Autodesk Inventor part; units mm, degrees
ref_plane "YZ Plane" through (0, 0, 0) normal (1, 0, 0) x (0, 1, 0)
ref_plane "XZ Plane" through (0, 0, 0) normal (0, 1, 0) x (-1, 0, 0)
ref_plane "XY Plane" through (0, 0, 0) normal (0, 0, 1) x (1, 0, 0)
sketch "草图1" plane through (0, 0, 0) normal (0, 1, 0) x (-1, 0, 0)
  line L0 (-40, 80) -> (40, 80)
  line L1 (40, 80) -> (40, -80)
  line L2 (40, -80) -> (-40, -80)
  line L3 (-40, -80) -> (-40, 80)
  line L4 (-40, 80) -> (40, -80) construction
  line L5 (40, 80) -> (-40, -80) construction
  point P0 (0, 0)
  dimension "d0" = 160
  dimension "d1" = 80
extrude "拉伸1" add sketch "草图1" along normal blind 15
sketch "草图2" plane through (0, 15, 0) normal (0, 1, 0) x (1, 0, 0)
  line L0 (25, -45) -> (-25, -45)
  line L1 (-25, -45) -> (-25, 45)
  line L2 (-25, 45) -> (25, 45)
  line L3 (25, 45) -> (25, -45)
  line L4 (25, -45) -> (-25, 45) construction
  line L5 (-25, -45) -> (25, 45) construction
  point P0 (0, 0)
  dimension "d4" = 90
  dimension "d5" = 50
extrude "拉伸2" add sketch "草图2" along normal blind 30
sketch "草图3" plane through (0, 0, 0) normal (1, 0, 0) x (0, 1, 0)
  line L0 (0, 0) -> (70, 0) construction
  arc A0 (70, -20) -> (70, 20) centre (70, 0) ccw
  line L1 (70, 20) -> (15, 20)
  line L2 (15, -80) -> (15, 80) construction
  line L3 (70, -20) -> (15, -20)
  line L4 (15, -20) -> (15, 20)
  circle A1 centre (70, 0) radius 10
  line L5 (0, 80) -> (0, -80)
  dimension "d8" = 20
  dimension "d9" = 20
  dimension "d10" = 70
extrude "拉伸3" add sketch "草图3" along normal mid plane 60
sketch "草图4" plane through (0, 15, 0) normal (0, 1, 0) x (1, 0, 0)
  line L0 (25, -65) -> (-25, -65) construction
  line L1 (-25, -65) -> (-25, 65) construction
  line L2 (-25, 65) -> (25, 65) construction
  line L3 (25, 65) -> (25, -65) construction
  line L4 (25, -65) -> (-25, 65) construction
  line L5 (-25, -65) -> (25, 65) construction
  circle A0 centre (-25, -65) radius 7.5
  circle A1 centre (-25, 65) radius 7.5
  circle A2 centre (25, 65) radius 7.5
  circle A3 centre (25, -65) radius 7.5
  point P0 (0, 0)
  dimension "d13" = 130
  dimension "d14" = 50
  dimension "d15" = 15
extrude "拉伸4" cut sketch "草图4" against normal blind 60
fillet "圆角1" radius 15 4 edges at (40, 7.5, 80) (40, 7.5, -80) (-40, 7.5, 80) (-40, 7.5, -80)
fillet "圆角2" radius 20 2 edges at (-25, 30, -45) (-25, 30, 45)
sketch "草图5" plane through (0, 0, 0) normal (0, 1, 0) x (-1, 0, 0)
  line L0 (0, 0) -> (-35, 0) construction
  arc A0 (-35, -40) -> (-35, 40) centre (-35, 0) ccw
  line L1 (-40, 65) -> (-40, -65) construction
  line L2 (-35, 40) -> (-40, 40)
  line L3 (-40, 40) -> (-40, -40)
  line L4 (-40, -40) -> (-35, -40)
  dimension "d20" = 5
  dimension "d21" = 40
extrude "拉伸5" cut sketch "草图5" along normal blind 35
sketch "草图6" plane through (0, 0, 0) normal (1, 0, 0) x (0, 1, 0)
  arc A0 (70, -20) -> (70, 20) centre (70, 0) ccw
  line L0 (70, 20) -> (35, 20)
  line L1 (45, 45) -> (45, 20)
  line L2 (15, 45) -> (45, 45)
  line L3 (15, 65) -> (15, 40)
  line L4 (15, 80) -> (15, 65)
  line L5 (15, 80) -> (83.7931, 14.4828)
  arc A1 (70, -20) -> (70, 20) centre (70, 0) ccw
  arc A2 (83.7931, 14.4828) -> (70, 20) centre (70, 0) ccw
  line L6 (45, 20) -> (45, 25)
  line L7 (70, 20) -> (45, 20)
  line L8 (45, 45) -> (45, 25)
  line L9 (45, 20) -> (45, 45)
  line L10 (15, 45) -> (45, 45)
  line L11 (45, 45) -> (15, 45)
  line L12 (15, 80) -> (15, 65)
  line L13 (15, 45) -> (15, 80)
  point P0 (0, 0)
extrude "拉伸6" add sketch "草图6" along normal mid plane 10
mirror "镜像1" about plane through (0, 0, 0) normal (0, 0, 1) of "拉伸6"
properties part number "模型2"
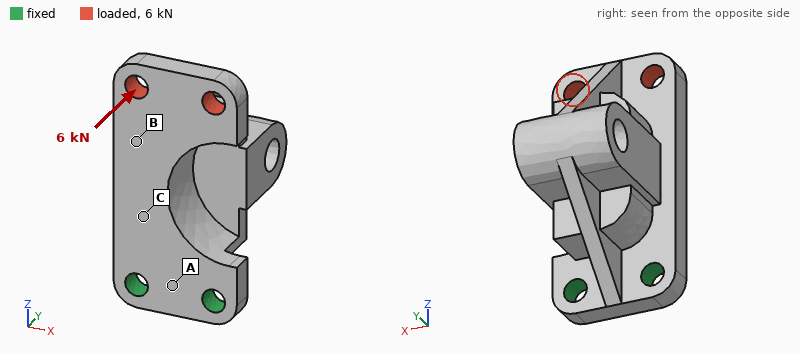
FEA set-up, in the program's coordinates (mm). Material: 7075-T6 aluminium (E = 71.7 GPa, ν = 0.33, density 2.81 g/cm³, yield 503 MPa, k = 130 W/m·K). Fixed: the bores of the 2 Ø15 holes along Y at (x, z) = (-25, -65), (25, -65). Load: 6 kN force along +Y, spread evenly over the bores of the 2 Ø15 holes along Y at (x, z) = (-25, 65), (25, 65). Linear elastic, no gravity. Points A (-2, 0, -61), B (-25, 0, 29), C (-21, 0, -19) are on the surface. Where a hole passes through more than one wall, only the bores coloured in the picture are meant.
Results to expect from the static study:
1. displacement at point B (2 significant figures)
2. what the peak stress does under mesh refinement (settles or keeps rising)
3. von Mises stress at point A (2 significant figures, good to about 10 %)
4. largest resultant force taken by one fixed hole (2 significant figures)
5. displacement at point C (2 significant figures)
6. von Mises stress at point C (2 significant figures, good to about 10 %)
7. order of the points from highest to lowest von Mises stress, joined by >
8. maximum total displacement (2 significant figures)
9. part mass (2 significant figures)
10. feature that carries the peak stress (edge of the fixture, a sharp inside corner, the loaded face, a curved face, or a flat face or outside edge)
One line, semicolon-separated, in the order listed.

0.64 mm; keeps rising; 73 MPa; 3.4 kN; 0.26 mm; 40 MPa; A > C > B; 1.2 mm; 960 g; edge of the fixture
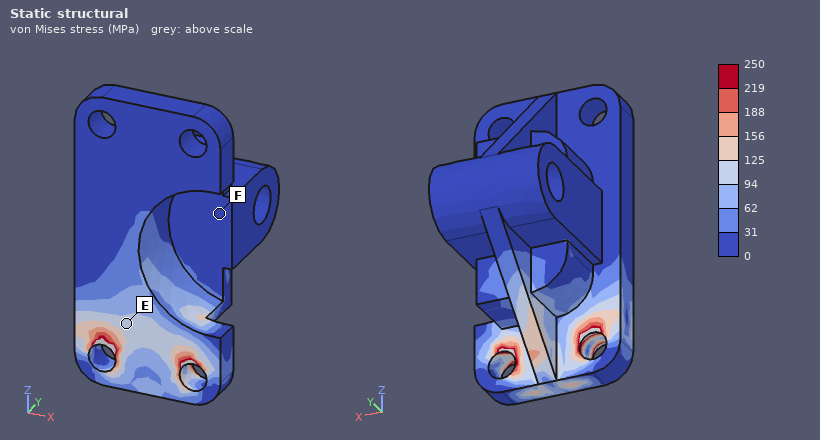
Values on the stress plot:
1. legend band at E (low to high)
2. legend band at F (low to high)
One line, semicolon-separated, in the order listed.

94 to 125 MPa; 0 to 31 MPa
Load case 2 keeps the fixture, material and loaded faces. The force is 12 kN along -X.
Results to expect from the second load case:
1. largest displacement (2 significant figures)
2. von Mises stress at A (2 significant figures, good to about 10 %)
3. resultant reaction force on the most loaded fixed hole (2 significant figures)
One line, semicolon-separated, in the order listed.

0.88 mm; 20 MPa; 30 kN
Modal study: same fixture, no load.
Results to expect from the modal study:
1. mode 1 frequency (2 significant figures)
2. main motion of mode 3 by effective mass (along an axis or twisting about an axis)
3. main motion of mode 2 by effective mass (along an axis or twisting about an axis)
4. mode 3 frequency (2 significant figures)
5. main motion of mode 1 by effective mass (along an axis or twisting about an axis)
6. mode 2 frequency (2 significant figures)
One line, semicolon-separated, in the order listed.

680 Hz; twisting about Z; along X; 1900 Hz; along Y; 1400 Hz
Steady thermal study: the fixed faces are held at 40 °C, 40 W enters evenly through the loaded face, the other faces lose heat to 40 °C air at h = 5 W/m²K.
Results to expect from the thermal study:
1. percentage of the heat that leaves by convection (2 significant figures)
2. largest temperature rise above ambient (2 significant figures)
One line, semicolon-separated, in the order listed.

8.9 %; 32 K
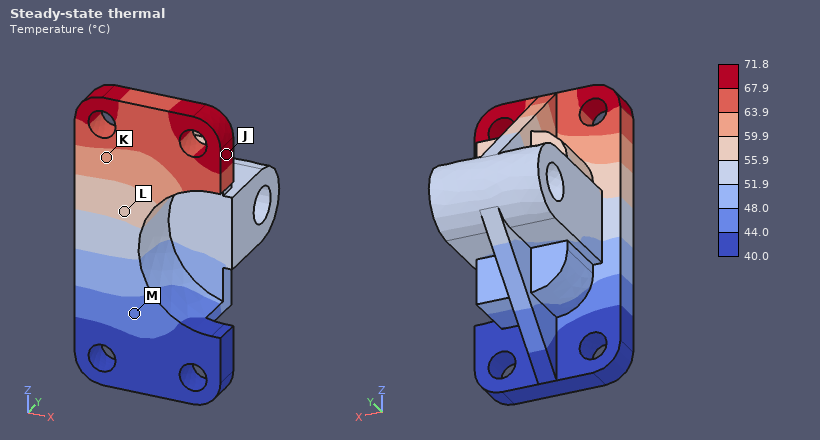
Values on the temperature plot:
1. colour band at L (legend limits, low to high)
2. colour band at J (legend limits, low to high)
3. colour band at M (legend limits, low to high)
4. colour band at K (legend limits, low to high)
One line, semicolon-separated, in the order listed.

55.9 to 59.9 °C; 67.9 to 71.8 °C; 44.0 to 48.0 °C; 59.9 to 63.9 °C
